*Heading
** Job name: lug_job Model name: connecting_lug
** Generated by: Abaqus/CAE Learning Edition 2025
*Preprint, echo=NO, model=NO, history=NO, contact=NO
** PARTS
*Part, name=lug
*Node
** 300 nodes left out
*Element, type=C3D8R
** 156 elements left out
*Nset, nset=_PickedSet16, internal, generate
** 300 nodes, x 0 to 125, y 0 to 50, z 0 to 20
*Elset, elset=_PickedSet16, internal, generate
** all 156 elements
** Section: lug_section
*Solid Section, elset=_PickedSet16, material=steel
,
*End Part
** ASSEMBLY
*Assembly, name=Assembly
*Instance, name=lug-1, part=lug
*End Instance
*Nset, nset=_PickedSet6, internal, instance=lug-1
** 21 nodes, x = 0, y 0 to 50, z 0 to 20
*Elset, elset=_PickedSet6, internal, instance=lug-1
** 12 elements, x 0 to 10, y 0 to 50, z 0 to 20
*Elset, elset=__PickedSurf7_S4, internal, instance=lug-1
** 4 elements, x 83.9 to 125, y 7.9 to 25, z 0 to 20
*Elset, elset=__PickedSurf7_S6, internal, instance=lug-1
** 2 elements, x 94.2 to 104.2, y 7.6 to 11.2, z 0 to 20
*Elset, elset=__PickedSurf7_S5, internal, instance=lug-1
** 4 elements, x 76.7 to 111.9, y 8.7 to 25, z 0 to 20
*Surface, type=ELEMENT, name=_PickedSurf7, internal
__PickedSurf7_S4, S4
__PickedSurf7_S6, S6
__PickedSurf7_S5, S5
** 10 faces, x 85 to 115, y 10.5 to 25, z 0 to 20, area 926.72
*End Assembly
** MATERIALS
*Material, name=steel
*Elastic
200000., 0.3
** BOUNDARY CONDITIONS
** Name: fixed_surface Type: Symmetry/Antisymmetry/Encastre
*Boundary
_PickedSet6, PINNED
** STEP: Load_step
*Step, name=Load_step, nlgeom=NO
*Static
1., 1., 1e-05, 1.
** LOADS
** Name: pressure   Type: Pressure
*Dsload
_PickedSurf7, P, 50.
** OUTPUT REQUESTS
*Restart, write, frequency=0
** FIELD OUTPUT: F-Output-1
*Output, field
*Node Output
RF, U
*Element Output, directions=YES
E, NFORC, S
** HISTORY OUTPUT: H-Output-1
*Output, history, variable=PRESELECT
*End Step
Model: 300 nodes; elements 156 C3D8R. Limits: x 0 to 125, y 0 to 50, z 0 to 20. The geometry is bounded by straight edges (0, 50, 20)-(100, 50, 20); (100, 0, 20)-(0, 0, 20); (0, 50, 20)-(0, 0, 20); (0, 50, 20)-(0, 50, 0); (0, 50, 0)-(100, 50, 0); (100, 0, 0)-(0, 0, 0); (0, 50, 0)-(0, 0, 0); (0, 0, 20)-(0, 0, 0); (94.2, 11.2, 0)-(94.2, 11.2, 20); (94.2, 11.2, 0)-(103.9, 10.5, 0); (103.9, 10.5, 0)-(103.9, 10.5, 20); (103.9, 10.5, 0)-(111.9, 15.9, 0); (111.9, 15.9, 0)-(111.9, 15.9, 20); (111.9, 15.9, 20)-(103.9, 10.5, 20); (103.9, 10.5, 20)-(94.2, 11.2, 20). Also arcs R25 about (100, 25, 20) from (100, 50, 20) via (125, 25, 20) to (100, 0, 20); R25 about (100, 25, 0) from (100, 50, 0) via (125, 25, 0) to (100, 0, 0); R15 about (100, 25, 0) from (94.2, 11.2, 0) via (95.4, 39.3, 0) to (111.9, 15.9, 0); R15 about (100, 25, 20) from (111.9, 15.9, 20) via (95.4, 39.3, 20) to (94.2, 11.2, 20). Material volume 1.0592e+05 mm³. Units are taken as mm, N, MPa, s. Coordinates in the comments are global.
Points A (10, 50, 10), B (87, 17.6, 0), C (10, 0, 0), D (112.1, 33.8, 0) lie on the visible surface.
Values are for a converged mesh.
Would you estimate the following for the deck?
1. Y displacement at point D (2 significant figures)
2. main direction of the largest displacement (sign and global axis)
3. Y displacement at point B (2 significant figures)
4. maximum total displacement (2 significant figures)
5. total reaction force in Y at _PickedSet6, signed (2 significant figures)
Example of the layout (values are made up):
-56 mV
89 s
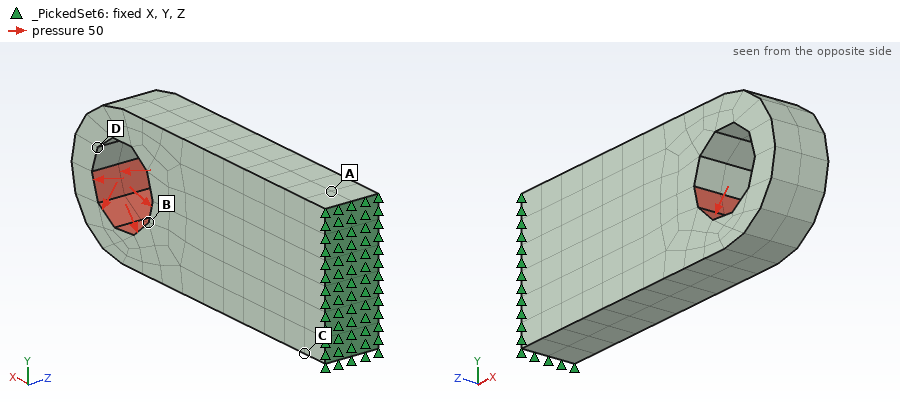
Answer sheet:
-0.37 mm
-Y
-0.23 mm
0.42 mm
30000 N
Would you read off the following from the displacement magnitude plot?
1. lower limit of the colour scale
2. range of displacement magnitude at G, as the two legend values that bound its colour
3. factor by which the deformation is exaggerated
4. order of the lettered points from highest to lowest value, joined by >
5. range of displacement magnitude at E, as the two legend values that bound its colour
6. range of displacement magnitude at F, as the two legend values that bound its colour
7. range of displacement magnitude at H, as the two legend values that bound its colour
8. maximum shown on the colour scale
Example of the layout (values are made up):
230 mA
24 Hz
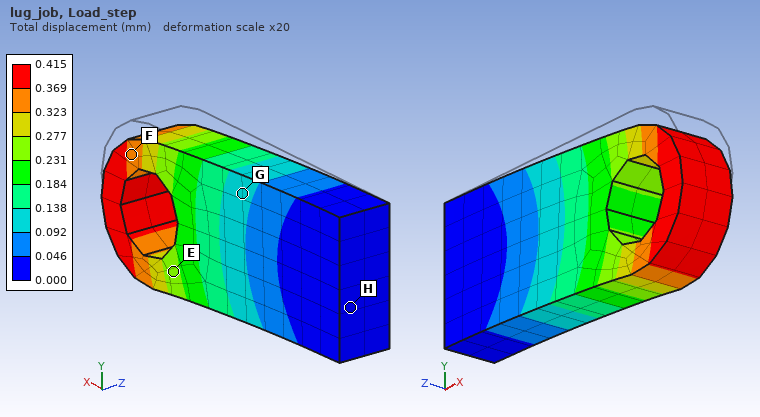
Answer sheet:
0.000 mm
0.092 to 0.138 mm
20
F > E > G > H
0.231 to 0.277 mm
0.323 to 0.369 mm
0.000 to 0.046 mm
0.415 mm
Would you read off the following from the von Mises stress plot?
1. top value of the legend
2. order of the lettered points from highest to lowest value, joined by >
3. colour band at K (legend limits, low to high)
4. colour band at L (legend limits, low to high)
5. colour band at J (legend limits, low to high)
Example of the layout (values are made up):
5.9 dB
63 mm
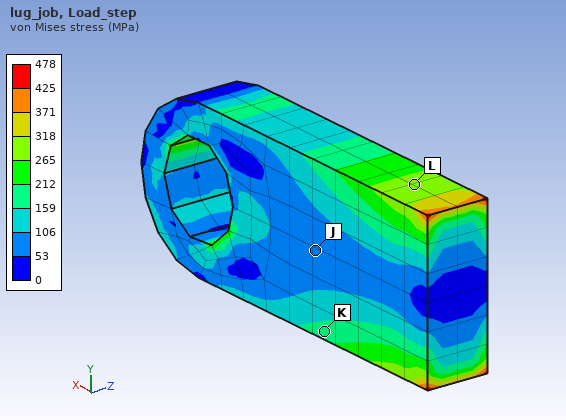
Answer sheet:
478 MPa
L > K > J
159 to 212 MPa
265 to 318 MPa
53 to 106 MPa
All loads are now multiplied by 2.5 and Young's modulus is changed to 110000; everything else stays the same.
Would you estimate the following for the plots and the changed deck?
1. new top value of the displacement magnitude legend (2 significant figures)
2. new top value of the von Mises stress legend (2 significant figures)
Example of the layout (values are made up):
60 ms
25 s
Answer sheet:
1.9 mm
1200 MPa
